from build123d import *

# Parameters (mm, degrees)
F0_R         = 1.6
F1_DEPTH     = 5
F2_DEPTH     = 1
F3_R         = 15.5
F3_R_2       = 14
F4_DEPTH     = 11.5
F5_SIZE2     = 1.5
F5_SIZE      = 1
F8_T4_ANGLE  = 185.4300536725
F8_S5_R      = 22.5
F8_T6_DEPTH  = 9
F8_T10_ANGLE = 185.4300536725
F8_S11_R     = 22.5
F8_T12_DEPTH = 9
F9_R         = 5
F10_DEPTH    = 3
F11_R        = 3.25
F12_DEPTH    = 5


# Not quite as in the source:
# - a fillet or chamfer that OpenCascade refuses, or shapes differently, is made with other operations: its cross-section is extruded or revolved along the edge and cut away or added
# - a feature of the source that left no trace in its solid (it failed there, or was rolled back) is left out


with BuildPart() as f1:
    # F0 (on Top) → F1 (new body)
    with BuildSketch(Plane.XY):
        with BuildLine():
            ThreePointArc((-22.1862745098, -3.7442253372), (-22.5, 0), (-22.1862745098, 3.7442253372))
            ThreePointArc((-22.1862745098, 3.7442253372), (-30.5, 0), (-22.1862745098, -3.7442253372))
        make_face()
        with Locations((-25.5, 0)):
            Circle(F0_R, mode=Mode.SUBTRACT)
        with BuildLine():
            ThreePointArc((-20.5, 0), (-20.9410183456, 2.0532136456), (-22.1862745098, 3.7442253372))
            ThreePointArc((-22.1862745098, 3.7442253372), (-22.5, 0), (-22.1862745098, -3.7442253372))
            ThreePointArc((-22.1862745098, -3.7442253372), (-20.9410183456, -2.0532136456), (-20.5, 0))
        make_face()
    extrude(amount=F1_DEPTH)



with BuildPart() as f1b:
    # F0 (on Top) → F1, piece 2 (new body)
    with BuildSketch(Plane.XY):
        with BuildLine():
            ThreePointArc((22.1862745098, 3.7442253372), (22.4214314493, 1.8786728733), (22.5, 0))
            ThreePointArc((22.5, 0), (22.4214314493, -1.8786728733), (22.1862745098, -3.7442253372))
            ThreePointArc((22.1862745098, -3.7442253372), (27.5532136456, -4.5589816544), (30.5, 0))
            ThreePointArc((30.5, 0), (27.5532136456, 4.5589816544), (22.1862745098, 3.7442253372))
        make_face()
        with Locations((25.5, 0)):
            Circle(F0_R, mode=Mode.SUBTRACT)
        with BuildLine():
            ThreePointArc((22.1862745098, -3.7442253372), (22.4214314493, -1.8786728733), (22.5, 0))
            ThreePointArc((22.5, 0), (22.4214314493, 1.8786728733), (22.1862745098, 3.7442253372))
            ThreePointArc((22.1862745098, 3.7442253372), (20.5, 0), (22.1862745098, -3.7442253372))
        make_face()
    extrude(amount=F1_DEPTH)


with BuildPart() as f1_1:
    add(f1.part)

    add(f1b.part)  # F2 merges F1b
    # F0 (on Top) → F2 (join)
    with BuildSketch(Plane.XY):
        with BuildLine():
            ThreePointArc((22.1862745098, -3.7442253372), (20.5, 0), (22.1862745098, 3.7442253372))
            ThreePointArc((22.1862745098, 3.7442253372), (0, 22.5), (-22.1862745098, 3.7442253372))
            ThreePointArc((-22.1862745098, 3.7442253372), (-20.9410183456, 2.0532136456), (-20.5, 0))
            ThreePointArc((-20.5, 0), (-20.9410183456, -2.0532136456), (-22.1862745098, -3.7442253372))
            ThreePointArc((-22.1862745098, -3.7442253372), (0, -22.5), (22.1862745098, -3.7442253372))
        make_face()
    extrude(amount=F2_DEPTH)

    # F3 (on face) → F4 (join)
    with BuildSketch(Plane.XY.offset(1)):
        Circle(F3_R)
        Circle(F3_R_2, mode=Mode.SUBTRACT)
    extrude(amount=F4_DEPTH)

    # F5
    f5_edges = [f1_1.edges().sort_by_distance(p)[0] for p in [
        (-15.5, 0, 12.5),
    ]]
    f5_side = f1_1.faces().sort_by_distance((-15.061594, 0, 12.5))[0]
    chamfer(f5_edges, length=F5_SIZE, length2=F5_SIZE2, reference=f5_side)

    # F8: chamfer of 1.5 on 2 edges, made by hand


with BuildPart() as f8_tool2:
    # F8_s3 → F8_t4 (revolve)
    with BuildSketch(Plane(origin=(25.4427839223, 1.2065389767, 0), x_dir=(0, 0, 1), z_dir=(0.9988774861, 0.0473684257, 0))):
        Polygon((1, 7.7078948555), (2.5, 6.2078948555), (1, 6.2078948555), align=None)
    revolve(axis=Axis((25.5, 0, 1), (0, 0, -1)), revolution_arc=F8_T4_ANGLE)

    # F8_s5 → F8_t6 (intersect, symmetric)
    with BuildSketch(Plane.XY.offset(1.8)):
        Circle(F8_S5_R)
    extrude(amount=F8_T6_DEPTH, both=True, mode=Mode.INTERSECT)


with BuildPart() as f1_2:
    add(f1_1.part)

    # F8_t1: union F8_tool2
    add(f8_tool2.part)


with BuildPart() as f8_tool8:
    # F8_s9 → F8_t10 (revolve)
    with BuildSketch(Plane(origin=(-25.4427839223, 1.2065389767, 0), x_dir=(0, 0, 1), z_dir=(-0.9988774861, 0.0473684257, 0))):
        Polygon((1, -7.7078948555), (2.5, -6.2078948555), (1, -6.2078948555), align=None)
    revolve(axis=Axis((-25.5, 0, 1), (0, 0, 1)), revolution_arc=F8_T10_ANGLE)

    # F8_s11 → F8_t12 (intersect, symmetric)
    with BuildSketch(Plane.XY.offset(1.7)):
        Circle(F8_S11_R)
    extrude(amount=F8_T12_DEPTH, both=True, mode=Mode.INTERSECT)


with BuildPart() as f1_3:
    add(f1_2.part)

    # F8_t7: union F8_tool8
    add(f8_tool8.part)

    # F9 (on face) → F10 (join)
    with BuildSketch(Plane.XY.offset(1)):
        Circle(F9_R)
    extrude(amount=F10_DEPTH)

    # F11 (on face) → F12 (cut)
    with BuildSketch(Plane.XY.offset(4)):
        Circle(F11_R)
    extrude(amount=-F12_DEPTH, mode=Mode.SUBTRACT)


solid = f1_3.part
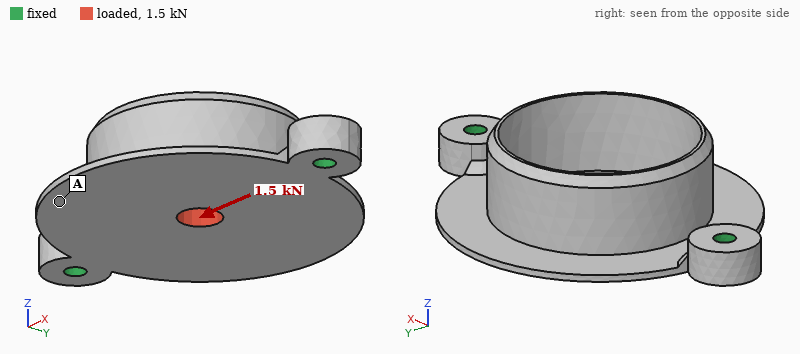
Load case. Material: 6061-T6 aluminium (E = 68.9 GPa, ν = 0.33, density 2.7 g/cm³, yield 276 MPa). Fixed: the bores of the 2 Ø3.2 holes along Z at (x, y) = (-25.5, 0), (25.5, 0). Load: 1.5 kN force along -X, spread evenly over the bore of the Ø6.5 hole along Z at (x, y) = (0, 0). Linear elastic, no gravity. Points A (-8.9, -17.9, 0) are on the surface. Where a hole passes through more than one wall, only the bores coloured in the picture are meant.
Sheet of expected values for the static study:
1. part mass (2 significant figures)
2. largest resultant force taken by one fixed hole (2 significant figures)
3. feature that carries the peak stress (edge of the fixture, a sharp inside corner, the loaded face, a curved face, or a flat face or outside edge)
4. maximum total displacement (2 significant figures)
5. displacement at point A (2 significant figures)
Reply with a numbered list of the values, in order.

1. 11 g
2. 750 N
3. a flat face or outside edge
4. 86 µm
5. 16 µm
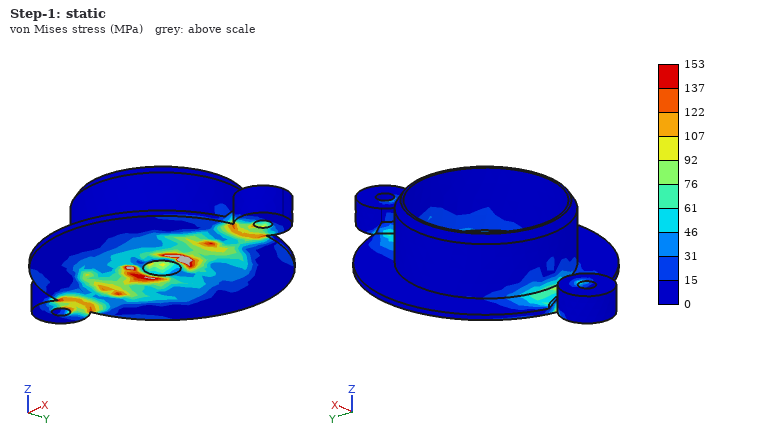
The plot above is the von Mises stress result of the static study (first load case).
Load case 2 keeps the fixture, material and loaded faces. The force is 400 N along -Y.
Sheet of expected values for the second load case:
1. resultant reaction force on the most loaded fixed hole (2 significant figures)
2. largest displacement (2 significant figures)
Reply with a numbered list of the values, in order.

1. 200 N
2. 99 µm
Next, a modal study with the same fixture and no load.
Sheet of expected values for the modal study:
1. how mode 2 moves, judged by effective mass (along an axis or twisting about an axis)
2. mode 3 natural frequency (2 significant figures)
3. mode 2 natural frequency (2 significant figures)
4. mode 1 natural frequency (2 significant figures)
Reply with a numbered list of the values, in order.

1. along Z
2. 6600 Hz
3. 3200 Hz
4. 1600 Hz
